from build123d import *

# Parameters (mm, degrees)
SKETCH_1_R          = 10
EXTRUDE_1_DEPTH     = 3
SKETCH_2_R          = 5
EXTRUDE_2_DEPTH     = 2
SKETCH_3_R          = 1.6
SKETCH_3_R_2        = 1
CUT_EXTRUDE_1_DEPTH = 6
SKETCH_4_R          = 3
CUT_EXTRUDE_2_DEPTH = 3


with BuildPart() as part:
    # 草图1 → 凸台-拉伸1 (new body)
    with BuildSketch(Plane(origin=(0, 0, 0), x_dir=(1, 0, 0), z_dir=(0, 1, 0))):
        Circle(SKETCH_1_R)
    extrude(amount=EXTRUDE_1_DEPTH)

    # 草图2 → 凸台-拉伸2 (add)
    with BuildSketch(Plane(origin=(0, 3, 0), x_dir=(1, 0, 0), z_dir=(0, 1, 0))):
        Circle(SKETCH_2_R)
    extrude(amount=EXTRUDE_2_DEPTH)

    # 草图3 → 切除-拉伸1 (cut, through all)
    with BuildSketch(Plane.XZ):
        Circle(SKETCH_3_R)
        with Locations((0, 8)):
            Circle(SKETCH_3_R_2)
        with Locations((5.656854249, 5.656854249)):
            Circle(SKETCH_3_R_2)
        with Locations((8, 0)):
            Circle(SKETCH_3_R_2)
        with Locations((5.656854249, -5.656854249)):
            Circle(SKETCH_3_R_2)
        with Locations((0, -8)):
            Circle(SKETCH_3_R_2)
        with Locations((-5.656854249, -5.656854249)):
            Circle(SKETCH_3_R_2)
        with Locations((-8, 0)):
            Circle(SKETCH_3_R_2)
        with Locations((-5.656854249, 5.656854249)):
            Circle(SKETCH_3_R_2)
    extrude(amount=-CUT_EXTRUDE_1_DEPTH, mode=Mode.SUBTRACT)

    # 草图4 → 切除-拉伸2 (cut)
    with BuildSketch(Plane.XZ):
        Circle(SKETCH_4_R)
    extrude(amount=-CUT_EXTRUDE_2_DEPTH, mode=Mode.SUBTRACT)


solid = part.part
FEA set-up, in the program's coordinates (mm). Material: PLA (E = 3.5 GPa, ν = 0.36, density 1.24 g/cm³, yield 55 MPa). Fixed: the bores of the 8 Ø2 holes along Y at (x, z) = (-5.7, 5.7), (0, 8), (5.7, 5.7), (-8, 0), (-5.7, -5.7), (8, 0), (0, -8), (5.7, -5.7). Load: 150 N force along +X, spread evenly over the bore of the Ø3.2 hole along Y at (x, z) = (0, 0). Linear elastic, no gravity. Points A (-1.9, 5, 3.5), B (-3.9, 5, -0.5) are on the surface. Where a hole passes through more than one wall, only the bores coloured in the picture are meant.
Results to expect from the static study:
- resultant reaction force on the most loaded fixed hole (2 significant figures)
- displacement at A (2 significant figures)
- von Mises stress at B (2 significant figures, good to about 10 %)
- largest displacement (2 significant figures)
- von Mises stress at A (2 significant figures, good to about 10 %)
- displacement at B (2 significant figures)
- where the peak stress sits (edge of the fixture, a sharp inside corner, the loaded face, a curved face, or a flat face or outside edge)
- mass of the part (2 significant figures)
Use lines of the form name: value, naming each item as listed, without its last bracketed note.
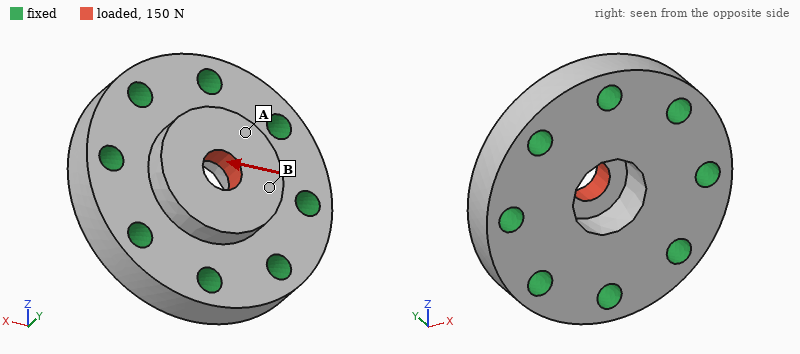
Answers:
resultant reaction force on the most loaded fixed hole: 34 N
displacement at A: 6.8 µm
von Mises stress at B: 5.0 MPa
largest displacement: 15 µm
von Mises stress at A: 2.6 MPa
displacement at B: 11 µm
where the peak stress sits: the loaded face
mass of the part: 1.1 g
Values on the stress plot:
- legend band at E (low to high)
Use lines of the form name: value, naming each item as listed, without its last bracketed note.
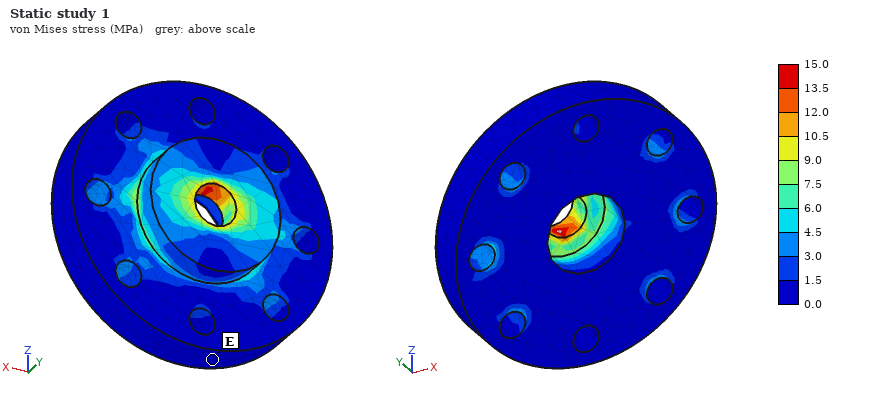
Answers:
legend band at E: 0.0 to 1.5 MPa
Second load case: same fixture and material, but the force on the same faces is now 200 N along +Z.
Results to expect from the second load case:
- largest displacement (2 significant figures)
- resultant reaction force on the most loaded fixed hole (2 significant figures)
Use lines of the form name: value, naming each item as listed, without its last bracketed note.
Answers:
largest displacement: 20 µm
resultant reaction force on the most loaded fixed hole: 45 N
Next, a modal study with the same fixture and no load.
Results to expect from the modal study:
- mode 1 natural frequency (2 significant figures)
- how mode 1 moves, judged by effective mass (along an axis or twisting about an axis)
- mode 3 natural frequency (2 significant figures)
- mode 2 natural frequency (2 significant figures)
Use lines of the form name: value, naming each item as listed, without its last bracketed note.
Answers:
mode 1 natural frequency: 35 kHz
how mode 1 moves, judged by effective mass: along Y
mode 3 natural frequency: 46 kHz
mode 2 natural frequency: 46 kHz
